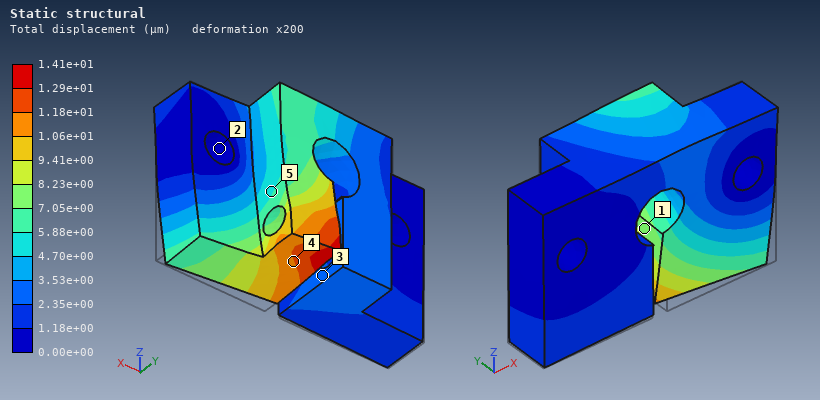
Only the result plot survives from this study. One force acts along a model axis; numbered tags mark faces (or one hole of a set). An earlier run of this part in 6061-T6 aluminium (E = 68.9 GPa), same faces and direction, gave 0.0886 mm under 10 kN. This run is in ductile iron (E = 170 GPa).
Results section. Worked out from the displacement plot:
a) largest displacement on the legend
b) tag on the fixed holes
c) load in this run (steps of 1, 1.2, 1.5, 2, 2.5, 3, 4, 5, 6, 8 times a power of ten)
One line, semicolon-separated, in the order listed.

1.41e+01 µm; 2; 4 kN
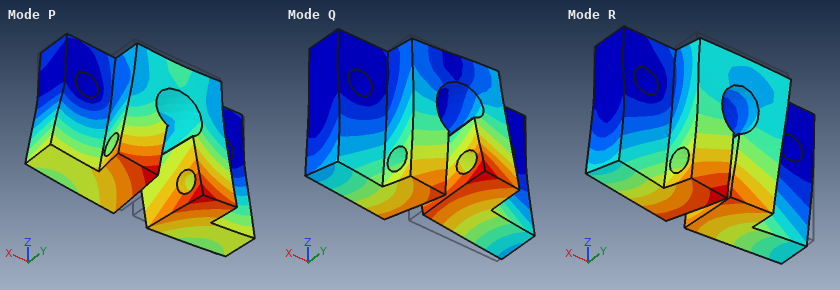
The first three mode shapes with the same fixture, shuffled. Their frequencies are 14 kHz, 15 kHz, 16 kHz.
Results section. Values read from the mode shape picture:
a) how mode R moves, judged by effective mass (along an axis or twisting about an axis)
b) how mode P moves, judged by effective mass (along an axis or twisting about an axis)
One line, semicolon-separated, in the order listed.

along Y; along Z
